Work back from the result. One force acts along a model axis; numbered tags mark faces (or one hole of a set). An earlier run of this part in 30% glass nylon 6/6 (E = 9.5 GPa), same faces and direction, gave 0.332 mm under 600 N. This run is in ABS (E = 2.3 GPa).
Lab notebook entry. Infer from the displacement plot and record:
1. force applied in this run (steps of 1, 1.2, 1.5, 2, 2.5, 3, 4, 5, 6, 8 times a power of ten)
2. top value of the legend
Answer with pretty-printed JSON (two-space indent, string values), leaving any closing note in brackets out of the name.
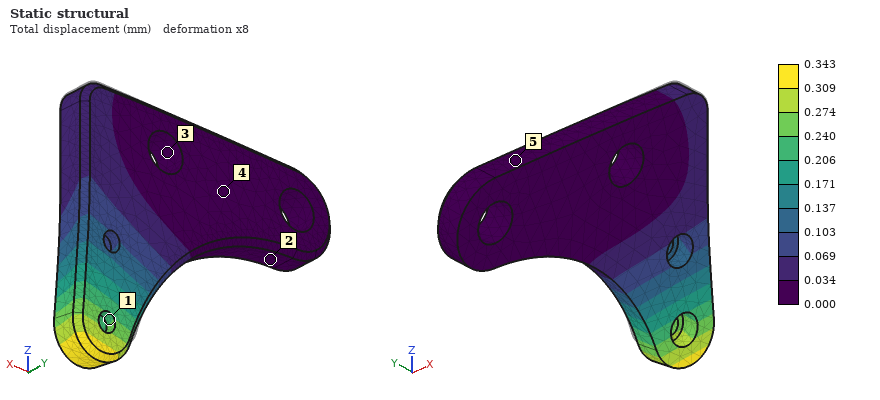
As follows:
{
  "force applied in this run": "150 N",
  "top value of the legend": "0.343 mm"
}
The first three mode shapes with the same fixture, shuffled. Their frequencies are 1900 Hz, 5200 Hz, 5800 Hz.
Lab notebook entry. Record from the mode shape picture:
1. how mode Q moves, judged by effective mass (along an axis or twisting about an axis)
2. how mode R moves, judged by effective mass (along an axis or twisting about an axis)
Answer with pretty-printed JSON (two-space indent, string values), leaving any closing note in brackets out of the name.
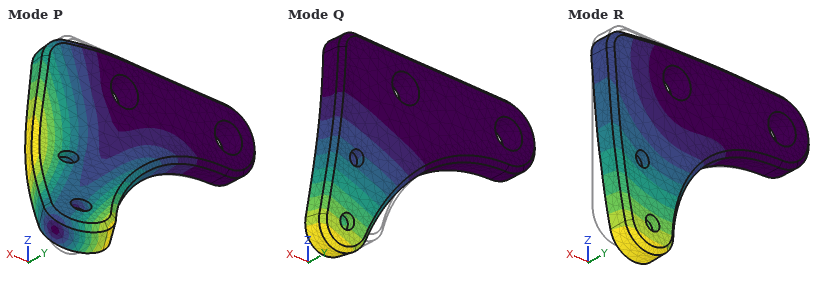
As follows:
{
  "how mode Q moves, judged by effective mass": "along Y",
  "how mode R moves, judged by effective mass": "along X"
}
